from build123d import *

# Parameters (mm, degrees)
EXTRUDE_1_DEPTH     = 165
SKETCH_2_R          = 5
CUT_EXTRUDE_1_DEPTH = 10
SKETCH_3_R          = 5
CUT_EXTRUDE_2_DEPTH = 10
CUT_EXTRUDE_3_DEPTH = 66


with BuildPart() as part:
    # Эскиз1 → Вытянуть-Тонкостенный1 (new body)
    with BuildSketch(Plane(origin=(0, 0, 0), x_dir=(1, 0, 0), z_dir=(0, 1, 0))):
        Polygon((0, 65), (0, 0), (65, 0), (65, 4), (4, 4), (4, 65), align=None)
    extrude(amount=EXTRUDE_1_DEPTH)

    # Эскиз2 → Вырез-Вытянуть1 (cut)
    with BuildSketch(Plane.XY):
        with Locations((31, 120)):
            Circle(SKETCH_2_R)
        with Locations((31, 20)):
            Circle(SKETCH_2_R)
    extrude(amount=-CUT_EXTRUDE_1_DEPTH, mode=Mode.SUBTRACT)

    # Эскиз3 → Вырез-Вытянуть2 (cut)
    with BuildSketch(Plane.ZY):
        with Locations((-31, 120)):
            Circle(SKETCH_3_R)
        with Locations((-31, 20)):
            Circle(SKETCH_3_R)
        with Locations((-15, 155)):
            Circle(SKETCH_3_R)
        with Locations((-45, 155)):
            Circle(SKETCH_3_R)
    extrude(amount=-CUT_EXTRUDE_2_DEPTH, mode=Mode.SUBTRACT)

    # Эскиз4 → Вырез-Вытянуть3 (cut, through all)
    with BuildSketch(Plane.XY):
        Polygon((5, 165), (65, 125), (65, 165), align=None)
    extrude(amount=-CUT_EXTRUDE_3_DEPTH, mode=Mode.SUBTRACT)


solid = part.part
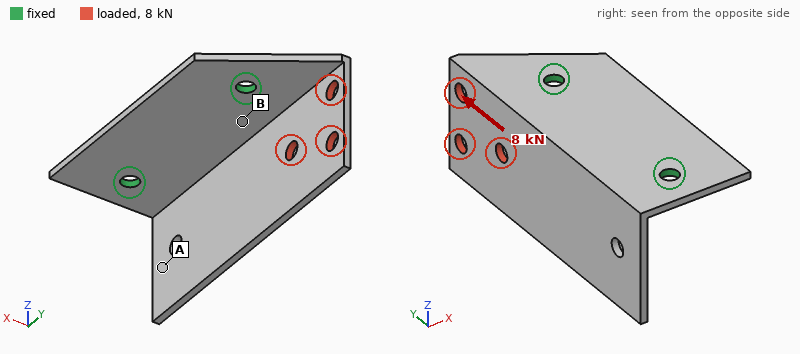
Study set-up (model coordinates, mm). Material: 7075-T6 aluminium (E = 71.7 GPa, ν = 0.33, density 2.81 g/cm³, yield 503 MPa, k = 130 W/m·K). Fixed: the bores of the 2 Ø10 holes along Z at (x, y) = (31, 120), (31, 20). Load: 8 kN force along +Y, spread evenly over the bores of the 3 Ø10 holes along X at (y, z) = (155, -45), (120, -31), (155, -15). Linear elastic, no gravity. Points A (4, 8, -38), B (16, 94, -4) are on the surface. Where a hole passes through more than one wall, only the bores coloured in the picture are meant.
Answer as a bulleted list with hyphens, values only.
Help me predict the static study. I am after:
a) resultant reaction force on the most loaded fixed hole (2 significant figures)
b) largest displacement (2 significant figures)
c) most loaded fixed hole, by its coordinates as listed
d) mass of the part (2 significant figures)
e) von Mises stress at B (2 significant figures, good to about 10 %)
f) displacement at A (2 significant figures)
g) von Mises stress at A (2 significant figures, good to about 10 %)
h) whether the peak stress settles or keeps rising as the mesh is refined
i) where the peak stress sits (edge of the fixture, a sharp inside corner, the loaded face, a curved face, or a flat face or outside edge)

- 5.4 kN
- 1.6 mm
- (31, 120)
- 210 g
- 110 MPa
- 0.95 mm
- 54 MPa
- keeps rising
- edge of the fixture
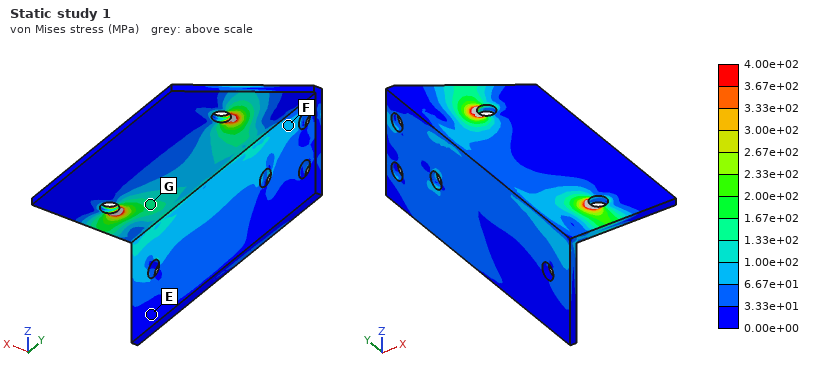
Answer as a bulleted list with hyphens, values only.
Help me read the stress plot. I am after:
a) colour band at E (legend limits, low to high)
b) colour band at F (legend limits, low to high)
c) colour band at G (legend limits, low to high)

- 0.00e+00 to 3.33e+01 MPa
- 6.67e+01 to 1.00e+02 MPa
- 1.33e+02 to 1.67e+02 MPa
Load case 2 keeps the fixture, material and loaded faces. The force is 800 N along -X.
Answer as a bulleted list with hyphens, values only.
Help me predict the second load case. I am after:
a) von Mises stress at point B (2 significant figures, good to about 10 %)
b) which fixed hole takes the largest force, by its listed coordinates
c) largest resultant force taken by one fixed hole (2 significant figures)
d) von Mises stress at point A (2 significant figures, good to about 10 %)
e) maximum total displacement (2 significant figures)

- 51 MPa
- (31, 120)
- 960 N
- 18 MPa
- 1.9 mm
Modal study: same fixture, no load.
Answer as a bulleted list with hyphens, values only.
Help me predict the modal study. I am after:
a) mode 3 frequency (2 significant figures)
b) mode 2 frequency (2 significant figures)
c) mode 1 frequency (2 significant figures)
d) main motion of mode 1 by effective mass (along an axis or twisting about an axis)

- 1400 Hz
- 760 Hz
- 460 Hz
- along X
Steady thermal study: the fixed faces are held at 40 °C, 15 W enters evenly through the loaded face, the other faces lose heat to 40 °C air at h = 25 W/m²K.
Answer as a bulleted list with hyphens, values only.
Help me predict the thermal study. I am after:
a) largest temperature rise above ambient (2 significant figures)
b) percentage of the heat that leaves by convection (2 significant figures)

- 21 K
- 36 %
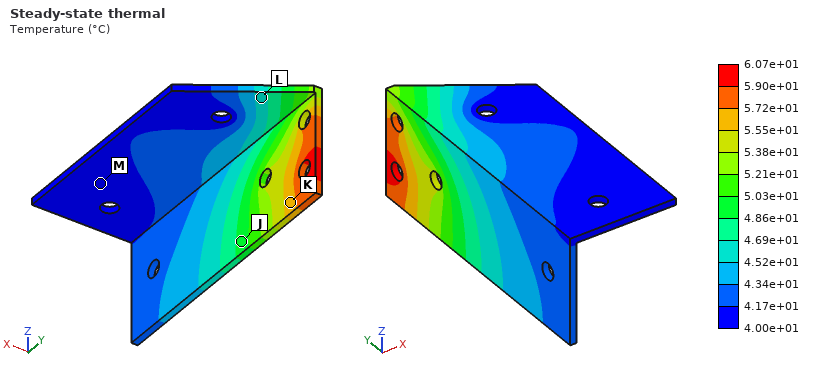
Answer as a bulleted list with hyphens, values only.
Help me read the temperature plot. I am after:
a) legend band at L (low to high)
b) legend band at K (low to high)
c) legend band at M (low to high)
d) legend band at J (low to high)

- 4.52e+01 to 4.69e+01 °C
- 5.55e+01 to 5.72e+01 °C
- 4.00e+01 to 4.17e+01 °C
- 4.86e+01 to 5.03e+01 °C
